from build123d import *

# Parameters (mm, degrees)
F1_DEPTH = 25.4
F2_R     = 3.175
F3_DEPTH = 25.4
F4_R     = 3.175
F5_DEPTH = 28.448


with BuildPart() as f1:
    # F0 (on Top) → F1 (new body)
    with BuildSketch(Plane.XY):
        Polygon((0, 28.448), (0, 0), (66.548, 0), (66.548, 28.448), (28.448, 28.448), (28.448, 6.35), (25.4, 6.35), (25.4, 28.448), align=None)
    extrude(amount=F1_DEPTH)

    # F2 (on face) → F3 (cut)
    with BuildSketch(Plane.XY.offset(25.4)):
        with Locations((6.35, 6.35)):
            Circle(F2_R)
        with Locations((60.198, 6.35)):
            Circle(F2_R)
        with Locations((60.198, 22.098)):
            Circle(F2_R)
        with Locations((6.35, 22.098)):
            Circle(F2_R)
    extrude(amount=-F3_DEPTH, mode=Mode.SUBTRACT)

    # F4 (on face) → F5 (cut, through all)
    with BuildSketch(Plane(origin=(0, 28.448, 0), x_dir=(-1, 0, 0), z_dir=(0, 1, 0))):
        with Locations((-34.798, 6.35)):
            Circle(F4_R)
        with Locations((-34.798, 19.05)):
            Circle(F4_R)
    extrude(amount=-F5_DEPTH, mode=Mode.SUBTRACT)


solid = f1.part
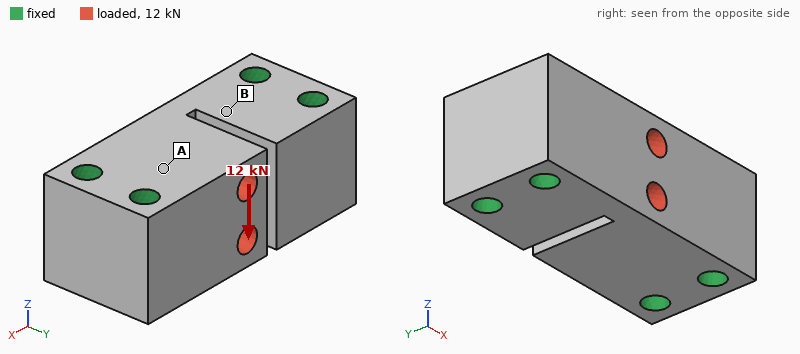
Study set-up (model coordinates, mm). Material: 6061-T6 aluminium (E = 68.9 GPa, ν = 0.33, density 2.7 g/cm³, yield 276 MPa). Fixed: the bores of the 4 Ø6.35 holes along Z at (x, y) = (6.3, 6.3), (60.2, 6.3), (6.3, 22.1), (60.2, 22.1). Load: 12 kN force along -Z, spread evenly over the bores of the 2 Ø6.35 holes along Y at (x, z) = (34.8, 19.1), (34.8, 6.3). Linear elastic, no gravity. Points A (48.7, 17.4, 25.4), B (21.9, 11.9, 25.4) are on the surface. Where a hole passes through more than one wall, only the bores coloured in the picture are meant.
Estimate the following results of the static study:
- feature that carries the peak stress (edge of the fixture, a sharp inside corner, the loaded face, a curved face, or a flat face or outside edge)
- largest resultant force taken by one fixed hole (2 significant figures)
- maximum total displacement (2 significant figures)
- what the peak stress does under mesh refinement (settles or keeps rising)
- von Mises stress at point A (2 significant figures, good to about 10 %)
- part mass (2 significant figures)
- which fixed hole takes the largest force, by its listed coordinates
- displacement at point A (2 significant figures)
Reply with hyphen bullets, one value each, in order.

- edge of the fixture
- 5.0 kN
- 38 µm
- keeps rising
- 30 MPa
- 110 g
- (60.2, 22.1)
- 11 µm
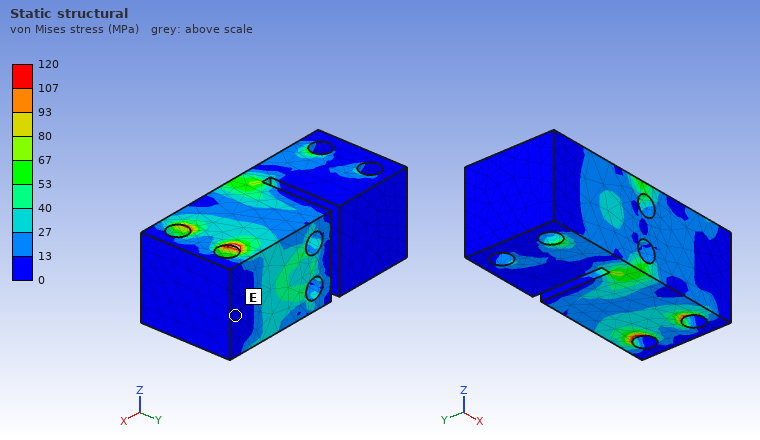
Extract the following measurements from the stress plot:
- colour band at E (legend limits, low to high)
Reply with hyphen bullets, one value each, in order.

- 0 to 13 MPa
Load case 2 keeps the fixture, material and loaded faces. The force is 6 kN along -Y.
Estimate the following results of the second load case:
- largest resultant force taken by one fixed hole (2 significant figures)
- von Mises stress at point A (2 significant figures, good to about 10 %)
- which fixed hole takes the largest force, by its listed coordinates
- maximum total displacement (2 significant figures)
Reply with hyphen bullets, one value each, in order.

- 4.8 kN
- 15 MPa
- (60.2, 22.1)
- 13 µm
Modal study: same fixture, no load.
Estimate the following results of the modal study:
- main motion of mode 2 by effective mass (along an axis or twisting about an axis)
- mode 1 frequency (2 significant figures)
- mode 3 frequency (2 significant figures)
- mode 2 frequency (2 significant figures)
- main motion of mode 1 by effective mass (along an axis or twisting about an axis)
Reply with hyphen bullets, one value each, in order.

- along Y
- 21 kHz
- 28 kHz
- 23 kHz
- along Z
